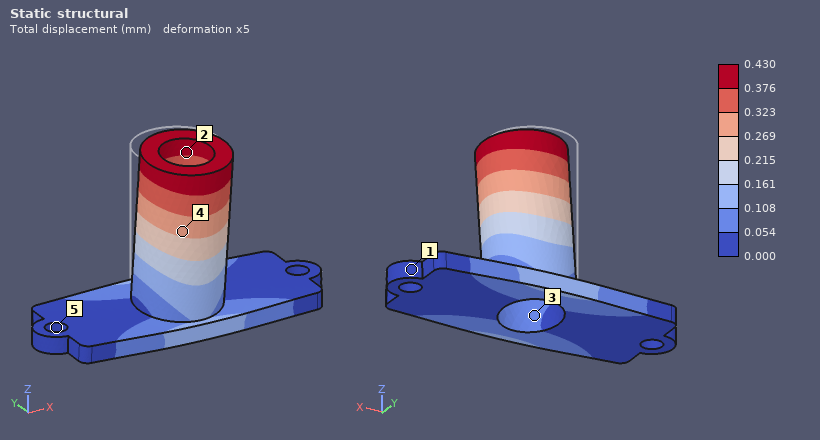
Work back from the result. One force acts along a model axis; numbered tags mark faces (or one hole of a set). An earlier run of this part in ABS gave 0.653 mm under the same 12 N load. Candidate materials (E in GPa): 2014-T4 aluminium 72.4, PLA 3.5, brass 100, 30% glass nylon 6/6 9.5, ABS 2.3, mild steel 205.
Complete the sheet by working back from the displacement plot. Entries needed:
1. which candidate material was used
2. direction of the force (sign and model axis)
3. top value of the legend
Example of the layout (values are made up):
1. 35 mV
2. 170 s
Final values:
1. PLA
2. -Y
3. 0.430 mm
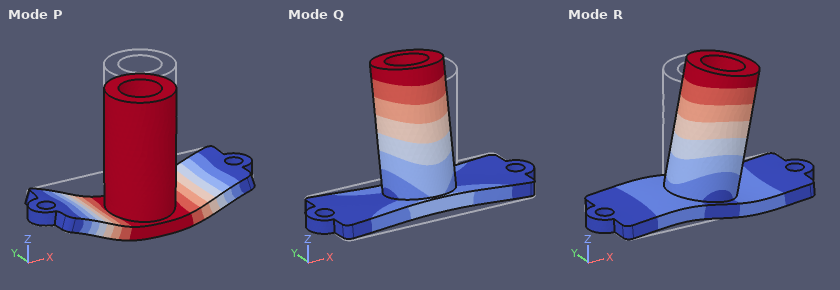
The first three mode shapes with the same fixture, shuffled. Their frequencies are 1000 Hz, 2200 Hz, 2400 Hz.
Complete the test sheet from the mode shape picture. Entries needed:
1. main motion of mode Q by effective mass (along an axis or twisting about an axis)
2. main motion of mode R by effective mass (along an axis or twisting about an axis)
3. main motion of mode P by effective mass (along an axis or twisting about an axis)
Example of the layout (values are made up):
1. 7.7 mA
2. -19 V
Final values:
1. along Y
2. along X
3. along Z
